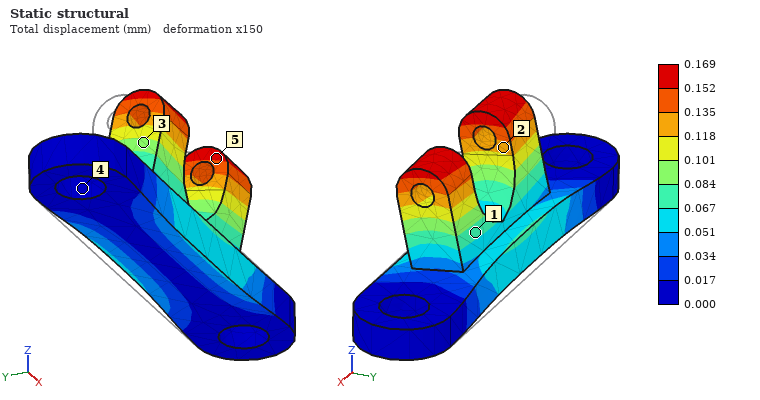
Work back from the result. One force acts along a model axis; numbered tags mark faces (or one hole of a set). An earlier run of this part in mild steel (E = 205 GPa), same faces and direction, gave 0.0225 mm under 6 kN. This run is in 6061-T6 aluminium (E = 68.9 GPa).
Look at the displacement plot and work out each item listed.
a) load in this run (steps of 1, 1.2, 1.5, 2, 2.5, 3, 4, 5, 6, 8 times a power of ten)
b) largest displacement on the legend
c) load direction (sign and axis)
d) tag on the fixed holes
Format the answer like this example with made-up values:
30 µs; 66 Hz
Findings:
15 kN; 0.169 mm; -Y; 4
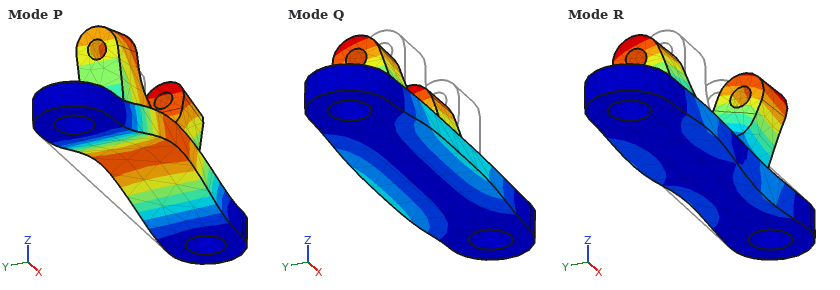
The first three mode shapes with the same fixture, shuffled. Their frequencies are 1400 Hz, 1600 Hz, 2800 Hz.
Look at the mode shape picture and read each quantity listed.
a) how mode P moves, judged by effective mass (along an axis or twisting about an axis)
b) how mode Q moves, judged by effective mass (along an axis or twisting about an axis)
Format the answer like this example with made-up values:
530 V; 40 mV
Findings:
along Z; along Y
